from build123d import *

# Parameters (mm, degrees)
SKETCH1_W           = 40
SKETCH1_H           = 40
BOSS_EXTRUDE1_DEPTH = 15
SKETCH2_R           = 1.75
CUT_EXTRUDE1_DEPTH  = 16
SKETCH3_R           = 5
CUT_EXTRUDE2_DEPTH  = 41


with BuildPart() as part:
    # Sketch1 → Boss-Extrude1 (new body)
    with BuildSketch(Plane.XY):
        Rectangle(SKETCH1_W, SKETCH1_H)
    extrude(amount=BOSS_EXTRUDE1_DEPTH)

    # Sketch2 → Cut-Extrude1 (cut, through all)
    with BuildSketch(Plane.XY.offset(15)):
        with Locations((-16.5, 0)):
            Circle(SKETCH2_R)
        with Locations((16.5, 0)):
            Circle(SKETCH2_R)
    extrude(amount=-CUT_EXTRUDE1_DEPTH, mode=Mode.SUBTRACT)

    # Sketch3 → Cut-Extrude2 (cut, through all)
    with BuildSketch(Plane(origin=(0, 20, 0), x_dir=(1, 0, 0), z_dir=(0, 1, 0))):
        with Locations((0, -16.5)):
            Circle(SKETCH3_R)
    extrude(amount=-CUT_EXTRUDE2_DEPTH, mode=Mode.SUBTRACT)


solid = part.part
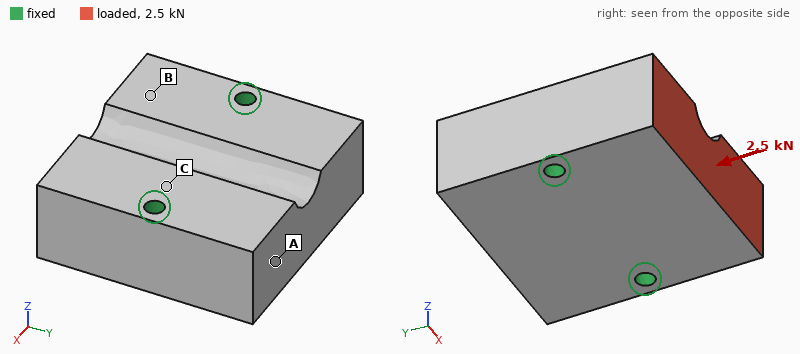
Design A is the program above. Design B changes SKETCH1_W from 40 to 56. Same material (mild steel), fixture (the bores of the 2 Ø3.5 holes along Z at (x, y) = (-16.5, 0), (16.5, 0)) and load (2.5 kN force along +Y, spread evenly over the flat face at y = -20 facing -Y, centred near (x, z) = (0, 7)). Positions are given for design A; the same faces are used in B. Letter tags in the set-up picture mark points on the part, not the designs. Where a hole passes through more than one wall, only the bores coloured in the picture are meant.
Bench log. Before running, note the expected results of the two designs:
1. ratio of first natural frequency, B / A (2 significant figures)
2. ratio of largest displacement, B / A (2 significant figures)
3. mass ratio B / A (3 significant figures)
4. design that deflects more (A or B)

0.92
0.70
1.42
A
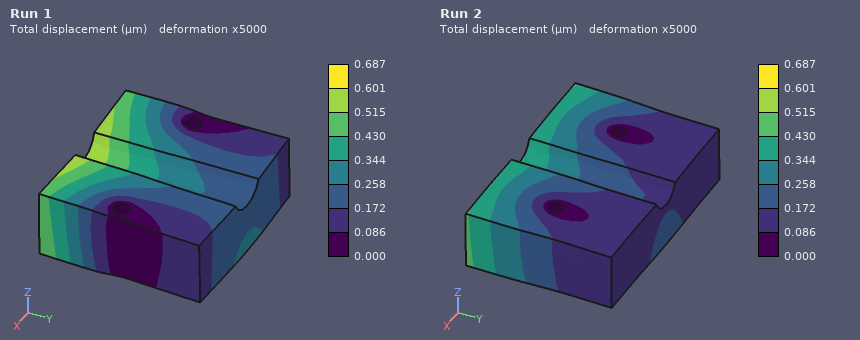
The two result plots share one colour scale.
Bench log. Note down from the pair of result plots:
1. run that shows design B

Run 2
